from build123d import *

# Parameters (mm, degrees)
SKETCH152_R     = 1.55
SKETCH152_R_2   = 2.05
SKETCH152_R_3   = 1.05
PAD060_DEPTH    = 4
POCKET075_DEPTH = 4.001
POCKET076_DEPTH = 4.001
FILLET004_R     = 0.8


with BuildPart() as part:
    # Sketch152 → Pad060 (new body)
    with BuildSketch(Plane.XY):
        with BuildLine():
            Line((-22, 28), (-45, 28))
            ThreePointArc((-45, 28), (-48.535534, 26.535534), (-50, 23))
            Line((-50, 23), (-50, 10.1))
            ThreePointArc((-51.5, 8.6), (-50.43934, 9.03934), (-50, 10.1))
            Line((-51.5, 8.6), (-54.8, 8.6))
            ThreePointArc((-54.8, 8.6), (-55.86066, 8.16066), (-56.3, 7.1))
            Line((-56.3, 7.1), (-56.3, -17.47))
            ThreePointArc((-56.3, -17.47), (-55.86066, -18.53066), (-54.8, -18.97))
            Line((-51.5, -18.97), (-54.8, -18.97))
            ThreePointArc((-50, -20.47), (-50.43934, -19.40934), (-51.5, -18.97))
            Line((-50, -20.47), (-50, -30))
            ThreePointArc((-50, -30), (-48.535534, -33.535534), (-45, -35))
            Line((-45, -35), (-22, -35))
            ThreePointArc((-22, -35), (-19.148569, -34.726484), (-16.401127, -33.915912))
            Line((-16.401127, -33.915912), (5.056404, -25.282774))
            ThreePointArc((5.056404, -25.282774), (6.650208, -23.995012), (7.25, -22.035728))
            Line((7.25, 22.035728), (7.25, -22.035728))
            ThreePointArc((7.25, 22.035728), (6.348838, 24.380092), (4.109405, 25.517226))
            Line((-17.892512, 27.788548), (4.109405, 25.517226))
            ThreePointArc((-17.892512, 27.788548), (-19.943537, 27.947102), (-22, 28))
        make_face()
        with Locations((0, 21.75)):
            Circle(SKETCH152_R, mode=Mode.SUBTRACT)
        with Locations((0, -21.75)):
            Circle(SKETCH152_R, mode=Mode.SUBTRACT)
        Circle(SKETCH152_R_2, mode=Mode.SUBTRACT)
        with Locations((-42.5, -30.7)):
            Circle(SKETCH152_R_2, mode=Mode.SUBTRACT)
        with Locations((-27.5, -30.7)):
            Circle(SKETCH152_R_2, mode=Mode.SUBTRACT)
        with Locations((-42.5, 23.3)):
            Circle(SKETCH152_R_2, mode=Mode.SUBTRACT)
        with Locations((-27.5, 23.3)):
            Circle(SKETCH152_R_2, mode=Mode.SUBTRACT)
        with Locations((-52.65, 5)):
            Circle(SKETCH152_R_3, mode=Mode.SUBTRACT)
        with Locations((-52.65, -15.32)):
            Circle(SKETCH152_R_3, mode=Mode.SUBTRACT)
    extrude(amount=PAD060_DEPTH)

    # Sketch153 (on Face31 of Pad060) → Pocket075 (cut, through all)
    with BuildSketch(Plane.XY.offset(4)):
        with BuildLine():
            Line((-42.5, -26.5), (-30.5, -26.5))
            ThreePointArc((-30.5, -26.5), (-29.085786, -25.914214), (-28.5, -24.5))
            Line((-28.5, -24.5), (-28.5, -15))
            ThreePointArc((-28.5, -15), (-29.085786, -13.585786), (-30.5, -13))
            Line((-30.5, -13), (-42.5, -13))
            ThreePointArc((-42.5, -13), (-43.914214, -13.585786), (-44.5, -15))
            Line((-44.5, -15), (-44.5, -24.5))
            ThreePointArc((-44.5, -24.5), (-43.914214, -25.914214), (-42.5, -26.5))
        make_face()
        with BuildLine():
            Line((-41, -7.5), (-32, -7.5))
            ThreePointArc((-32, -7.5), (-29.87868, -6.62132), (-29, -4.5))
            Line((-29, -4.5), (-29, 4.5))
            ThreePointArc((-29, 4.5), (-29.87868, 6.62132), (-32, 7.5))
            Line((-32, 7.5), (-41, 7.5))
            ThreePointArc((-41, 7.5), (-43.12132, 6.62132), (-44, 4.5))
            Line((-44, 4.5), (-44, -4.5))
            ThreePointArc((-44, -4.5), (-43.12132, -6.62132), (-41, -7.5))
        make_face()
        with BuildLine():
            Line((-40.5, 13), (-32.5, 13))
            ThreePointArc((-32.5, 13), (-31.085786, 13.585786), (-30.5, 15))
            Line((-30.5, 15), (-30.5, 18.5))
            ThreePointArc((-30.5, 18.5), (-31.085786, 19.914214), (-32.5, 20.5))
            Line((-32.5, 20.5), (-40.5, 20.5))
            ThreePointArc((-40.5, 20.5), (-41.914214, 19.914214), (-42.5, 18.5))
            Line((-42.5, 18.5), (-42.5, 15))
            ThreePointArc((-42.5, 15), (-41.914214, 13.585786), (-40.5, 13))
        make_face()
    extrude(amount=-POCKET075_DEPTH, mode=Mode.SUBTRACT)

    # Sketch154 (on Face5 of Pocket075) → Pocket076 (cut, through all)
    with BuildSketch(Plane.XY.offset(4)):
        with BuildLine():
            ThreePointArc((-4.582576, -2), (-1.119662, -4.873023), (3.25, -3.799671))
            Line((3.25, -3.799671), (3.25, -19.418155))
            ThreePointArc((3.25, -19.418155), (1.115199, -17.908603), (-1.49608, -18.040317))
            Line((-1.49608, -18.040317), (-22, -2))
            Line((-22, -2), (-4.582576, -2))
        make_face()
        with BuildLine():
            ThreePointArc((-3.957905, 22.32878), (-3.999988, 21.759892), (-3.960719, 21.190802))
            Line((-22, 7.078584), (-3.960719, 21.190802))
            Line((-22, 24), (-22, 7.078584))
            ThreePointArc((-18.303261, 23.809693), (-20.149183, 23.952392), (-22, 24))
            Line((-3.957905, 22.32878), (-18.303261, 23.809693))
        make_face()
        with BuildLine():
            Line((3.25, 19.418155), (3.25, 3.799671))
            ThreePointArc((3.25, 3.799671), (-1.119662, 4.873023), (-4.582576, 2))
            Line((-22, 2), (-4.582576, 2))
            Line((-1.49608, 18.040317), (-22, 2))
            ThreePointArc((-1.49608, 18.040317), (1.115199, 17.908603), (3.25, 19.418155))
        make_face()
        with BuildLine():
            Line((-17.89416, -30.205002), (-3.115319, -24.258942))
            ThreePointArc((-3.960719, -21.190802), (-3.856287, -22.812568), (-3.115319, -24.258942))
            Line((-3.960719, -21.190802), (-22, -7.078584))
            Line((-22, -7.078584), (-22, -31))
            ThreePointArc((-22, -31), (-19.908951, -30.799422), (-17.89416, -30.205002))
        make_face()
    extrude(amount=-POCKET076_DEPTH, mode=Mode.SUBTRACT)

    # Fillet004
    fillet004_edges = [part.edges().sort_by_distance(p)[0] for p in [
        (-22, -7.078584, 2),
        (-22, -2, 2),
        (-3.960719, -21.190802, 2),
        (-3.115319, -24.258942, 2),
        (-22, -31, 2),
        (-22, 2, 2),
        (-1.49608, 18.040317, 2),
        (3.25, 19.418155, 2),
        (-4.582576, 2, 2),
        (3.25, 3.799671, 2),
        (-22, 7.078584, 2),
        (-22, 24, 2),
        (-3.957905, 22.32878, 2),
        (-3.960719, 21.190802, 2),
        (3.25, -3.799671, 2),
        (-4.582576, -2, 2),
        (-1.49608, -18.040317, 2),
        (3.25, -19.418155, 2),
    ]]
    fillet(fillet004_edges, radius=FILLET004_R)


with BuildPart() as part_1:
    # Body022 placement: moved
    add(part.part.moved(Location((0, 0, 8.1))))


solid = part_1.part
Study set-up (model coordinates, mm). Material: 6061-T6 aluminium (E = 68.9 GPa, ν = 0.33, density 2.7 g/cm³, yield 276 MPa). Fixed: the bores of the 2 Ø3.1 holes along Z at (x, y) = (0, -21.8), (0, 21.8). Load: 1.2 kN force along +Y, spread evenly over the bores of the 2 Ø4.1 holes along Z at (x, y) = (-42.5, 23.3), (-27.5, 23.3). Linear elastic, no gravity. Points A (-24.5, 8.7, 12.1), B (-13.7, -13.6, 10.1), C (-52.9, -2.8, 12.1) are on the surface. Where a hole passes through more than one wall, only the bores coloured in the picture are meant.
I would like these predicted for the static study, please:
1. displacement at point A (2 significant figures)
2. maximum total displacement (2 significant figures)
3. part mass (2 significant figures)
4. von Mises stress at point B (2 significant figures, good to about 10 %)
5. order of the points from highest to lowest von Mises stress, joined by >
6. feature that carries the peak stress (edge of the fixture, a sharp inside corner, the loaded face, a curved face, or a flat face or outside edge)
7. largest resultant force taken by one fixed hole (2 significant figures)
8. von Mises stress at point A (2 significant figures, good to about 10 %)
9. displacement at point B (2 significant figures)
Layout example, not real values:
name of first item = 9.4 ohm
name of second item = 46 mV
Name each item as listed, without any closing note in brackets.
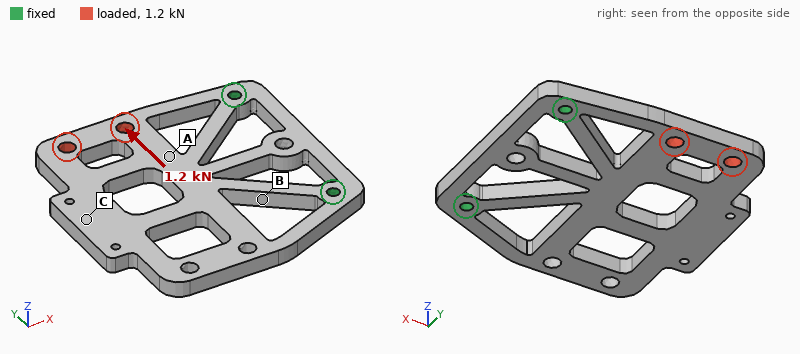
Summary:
displacement at point A = 42 µm
maximum total displacement = 76 µm
part mass = 23 g
von Mises stress at point B = 62 MPa
order of the points from highest to lowest von Mises stress, joined by > = B > A > C
feature that carries the peak stress = a curved face
largest resultant force taken by one fixed hole = 1.1 kN
von Mises stress at point A = 23 MPa
displacement at point B = 22 µm
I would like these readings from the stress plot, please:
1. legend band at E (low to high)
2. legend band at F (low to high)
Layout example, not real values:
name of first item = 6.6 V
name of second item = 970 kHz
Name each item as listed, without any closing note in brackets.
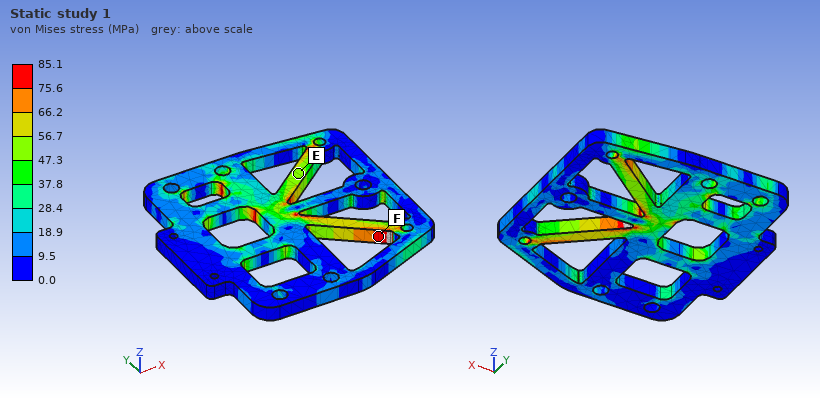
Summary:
legend band at E = 47.3 to 56.7 MPa
legend band at F = 75.6 to 85.1 MPa
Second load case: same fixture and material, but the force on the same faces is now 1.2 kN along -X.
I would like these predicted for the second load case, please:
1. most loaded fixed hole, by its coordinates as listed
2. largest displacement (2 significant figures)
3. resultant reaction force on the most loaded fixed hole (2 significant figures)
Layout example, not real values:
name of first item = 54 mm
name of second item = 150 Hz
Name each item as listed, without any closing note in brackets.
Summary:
most loaded fixed hole, by its coordinates as listed = (0, 21.8)
largest displacement = 35 µm
resultant reaction force on the most loaded fixed hole = 1.2 kN
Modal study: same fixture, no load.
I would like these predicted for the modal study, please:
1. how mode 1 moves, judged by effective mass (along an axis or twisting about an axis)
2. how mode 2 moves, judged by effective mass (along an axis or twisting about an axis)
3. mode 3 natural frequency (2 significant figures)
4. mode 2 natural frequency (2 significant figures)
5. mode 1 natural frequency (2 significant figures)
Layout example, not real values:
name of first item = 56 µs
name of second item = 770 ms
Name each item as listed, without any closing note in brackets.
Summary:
how mode 1 moves, judged by effective mass = along Z
how mode 2 moves, judged by effective mass = twisting about X
mode 3 natural frequency = 4300 Hz
mode 2 natural frequency = 1900 Hz
mode 1 natural frequency = 700 Hz
